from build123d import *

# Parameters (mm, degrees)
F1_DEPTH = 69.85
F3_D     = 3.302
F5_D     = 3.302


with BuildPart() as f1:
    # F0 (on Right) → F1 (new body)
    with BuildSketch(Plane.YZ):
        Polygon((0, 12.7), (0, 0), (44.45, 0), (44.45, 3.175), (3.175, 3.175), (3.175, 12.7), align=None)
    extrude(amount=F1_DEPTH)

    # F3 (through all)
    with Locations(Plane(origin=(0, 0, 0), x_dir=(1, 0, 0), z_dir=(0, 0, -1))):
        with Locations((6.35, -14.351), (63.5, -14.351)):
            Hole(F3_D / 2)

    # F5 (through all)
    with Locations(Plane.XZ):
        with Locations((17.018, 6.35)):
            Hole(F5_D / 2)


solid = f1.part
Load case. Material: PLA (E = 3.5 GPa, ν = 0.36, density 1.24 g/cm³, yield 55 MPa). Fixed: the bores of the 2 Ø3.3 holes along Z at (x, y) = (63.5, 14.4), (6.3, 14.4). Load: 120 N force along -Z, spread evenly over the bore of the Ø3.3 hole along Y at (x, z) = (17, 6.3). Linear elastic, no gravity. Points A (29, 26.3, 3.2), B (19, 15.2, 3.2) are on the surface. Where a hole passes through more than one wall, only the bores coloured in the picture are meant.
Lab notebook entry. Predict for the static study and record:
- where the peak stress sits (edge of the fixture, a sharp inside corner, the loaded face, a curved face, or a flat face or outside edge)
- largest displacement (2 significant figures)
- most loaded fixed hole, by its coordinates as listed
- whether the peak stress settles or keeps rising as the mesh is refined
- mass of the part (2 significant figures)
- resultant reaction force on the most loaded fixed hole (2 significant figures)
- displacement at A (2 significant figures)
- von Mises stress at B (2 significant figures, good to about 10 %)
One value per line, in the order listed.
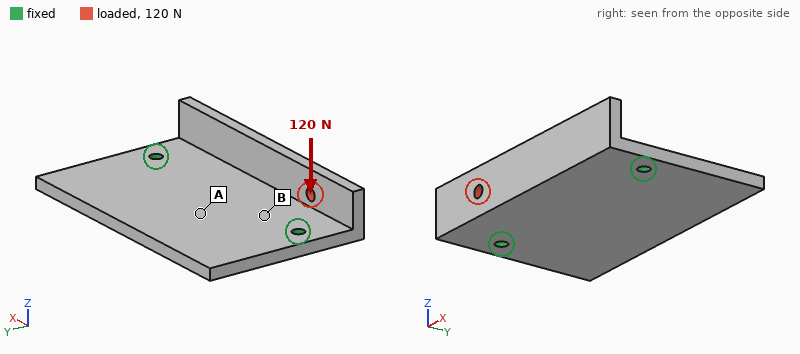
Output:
edge of the fixture
0.57 mm
(6.3, 14.4)
keeps rising
15 g
100 N
0.10 mm
6.3 MPa
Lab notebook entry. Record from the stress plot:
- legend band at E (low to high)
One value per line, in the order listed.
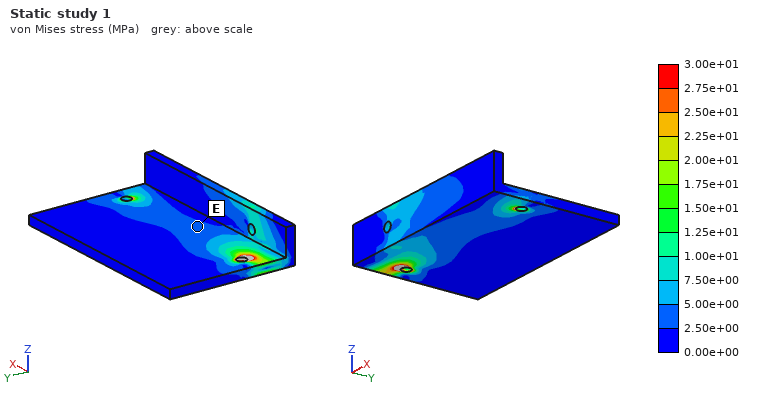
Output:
2.50e+00 to 5.00e+00 MPa
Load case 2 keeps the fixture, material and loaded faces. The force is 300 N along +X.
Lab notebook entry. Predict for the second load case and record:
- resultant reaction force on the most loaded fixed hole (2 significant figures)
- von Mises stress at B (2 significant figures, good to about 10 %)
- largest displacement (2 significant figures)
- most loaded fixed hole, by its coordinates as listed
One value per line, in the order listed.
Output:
190 N
2.8 MPa
0.15 mm
(6.3, 14.4)
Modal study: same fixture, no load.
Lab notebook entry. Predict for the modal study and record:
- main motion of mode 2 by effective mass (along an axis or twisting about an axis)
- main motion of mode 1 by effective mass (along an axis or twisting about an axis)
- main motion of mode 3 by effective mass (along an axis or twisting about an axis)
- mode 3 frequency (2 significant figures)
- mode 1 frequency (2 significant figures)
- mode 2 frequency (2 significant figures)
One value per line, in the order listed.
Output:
twisting about Y
along Z
along Z
1500 Hz
680 Hz
1300 Hz
